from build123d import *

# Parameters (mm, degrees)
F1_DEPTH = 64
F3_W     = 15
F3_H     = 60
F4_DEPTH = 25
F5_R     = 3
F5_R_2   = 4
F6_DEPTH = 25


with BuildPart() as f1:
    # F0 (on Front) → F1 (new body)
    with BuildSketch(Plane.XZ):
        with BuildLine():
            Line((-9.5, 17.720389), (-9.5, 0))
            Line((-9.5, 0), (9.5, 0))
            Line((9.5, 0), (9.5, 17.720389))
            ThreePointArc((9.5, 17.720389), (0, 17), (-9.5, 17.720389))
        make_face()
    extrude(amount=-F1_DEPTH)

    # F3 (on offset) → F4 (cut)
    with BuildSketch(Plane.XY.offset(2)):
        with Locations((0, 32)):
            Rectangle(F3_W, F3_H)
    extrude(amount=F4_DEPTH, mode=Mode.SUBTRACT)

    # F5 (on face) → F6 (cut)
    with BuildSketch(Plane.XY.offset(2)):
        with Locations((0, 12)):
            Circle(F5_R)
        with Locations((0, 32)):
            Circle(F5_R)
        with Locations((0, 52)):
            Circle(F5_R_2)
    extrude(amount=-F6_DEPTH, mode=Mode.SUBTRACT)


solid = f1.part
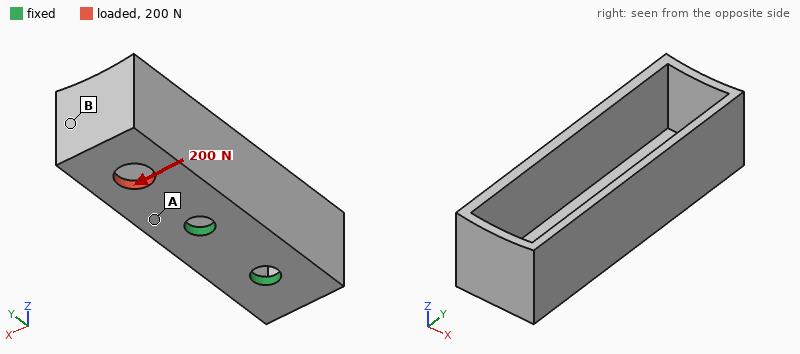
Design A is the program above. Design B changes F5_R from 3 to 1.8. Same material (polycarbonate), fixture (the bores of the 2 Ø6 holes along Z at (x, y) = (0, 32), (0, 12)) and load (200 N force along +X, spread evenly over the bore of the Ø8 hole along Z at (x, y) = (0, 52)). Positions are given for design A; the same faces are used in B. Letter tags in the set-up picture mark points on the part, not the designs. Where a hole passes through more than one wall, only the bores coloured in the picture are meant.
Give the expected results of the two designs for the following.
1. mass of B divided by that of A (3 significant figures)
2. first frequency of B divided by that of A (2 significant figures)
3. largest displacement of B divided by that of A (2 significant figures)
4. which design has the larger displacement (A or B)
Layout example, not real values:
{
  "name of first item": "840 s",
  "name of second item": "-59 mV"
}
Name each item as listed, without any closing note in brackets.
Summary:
{
  "mass of B divided by that of A": "1.01",
  "first frequency of B divided by that of A": "0.88",
  "largest displacement of B divided by that of A": "1.2",
  "which design has the larger displacement": "B"
}
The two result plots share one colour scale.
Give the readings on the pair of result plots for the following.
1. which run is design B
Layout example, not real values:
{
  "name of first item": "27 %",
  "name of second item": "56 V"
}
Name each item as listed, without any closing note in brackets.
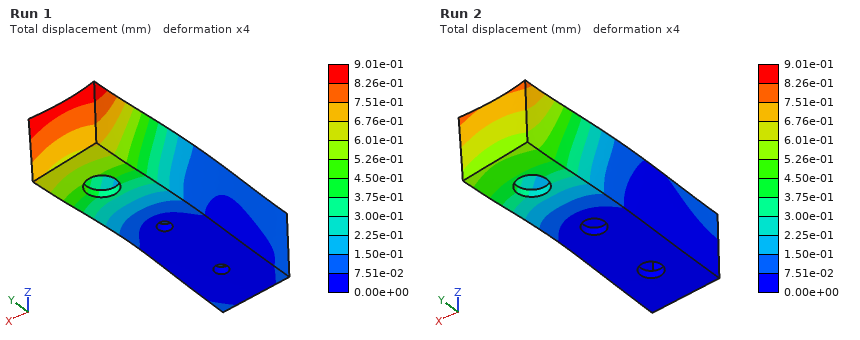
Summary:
{
  "which run is design B": "Run 1"
}
